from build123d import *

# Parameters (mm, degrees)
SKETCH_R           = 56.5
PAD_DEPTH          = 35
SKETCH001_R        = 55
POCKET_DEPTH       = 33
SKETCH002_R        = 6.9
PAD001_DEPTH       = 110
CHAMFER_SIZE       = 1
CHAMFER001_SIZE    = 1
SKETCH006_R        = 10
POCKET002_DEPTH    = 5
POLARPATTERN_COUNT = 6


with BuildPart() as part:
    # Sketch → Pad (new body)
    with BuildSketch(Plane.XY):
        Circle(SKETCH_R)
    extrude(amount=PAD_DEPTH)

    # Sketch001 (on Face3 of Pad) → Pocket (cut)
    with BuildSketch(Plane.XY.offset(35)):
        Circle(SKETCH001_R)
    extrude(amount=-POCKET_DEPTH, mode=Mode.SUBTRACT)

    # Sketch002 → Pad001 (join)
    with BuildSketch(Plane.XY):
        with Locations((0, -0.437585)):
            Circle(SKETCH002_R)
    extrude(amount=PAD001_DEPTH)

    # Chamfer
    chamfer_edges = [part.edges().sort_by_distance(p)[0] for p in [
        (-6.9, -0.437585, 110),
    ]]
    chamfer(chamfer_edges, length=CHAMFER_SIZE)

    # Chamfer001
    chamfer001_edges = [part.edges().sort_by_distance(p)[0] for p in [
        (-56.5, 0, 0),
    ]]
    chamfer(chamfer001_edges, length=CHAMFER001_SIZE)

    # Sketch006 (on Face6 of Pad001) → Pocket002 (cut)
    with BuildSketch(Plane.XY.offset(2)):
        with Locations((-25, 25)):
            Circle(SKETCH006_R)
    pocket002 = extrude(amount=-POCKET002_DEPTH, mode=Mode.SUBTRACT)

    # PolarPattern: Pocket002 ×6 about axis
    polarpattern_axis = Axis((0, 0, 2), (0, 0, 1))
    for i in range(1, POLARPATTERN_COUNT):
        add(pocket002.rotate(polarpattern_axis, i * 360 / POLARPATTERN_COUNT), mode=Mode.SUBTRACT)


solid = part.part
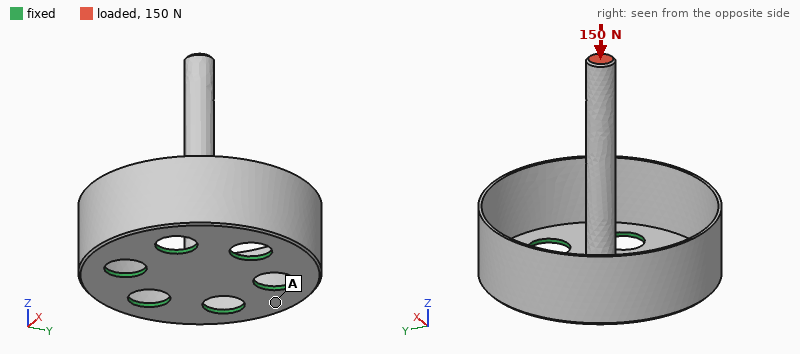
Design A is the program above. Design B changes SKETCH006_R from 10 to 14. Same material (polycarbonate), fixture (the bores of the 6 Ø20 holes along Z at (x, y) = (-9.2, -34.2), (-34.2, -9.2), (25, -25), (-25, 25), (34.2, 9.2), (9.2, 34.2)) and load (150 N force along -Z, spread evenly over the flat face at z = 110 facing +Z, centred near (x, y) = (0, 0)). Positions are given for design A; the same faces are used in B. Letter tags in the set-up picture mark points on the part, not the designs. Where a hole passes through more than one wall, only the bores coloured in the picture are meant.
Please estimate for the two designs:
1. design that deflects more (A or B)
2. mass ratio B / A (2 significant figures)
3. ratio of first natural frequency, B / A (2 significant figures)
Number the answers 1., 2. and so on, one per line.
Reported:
1. A
2. 0.93
3. 1.1
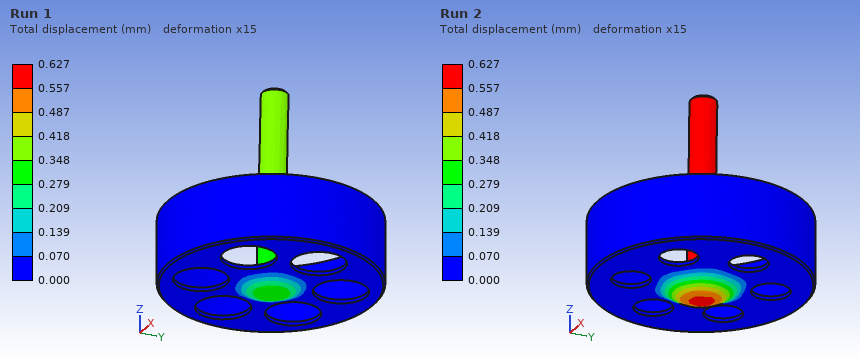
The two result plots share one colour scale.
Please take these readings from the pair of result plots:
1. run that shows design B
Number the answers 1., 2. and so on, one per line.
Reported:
1. Run 1
